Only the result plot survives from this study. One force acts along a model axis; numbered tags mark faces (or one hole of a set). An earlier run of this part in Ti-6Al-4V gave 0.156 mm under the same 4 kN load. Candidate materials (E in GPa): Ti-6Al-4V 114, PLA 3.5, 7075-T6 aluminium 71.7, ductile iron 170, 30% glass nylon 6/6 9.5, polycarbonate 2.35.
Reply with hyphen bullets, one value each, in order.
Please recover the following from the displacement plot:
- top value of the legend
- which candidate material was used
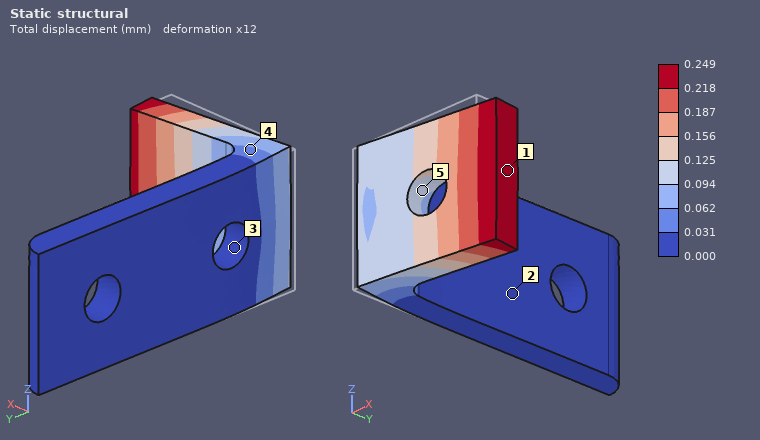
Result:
- 0.249 mm
- 7075-T6 aluminium
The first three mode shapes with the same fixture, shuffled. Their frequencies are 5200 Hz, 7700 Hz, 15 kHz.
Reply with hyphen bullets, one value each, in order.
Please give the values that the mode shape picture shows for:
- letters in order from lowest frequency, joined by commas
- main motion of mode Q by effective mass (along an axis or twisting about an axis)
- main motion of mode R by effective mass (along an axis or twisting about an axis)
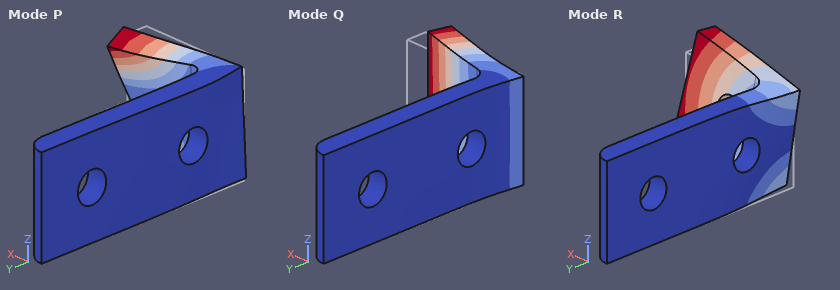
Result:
- Q, R, P
- along Y
- along Z
